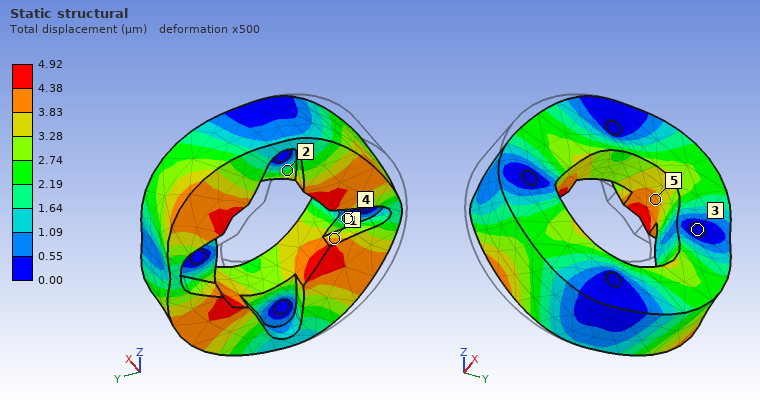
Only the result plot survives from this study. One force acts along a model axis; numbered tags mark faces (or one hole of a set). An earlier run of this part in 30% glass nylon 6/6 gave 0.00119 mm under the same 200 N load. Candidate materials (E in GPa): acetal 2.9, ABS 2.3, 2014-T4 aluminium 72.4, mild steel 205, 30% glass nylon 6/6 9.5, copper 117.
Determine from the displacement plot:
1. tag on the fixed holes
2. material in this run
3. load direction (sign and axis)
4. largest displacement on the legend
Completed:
3
ABS
+Y
4.92 µm
